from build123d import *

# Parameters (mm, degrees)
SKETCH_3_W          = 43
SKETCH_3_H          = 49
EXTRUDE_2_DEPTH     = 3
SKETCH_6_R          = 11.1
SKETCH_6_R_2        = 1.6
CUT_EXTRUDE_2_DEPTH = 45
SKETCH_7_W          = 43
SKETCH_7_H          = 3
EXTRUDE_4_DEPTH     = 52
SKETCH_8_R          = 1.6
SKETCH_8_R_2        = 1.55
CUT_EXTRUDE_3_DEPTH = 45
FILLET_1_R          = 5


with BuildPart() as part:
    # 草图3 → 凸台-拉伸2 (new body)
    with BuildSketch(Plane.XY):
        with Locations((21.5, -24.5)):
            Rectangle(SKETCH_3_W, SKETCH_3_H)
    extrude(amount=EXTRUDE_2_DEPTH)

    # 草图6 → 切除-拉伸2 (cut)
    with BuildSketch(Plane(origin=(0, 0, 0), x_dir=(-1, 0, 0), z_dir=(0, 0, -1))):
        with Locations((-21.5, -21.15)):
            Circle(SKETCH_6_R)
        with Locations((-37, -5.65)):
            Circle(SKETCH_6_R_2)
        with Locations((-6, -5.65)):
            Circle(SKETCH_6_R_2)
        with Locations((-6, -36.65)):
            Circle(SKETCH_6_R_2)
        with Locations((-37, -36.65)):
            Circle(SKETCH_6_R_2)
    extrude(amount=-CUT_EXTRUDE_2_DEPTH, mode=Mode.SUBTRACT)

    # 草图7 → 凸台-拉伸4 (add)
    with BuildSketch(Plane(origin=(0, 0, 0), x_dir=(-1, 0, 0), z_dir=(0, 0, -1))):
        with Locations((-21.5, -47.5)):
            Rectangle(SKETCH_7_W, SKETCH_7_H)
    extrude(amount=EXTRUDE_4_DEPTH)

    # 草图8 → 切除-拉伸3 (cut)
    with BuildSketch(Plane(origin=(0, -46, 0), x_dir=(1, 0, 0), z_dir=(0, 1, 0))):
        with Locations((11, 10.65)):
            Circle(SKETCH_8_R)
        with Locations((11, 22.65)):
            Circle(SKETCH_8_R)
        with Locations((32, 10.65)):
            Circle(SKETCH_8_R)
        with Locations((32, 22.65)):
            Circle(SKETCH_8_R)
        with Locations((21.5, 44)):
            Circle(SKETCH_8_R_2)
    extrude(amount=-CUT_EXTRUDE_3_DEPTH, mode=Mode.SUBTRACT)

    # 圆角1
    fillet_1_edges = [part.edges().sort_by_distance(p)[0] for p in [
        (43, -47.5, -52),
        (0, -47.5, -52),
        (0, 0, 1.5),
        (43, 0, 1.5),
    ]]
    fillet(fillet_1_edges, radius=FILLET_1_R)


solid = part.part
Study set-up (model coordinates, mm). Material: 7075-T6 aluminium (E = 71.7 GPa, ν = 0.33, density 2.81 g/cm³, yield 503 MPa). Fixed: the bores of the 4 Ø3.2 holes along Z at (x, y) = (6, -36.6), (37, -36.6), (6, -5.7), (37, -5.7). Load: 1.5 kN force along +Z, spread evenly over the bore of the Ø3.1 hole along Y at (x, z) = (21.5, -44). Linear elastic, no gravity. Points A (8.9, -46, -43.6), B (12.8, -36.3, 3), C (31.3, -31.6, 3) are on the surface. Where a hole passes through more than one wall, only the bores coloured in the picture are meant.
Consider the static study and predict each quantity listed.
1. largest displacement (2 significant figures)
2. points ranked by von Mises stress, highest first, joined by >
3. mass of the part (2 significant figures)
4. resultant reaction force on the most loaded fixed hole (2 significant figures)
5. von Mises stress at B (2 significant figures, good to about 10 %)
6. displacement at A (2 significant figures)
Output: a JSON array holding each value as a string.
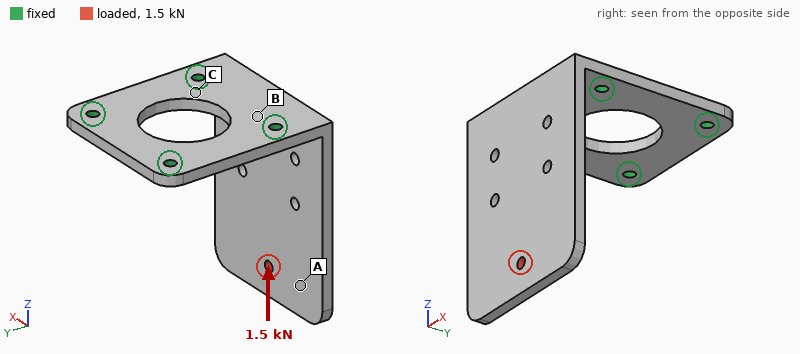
["0.78 mm", "B > C > A", "33 g", "790 N", "98 MPa", "0.65 mm"]
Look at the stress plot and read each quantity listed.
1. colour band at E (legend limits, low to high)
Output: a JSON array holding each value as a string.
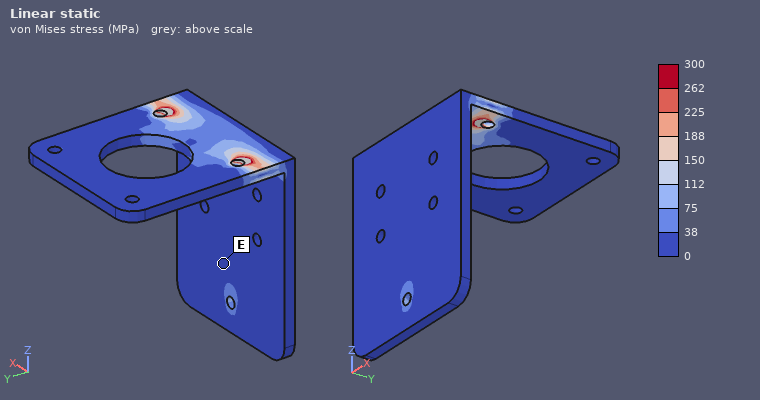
["0 to 38 MPa"]
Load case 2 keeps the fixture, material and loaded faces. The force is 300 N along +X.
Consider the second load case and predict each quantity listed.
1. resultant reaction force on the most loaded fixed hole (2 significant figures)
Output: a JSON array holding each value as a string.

["470 N"]
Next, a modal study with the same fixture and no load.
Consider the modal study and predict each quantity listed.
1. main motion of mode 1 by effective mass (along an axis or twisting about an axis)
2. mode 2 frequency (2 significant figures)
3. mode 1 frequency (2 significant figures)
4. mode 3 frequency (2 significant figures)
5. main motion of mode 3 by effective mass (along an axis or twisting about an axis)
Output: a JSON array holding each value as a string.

["along Y", "2000 Hz", "650 Hz", "2800 Hz", "along X"]
